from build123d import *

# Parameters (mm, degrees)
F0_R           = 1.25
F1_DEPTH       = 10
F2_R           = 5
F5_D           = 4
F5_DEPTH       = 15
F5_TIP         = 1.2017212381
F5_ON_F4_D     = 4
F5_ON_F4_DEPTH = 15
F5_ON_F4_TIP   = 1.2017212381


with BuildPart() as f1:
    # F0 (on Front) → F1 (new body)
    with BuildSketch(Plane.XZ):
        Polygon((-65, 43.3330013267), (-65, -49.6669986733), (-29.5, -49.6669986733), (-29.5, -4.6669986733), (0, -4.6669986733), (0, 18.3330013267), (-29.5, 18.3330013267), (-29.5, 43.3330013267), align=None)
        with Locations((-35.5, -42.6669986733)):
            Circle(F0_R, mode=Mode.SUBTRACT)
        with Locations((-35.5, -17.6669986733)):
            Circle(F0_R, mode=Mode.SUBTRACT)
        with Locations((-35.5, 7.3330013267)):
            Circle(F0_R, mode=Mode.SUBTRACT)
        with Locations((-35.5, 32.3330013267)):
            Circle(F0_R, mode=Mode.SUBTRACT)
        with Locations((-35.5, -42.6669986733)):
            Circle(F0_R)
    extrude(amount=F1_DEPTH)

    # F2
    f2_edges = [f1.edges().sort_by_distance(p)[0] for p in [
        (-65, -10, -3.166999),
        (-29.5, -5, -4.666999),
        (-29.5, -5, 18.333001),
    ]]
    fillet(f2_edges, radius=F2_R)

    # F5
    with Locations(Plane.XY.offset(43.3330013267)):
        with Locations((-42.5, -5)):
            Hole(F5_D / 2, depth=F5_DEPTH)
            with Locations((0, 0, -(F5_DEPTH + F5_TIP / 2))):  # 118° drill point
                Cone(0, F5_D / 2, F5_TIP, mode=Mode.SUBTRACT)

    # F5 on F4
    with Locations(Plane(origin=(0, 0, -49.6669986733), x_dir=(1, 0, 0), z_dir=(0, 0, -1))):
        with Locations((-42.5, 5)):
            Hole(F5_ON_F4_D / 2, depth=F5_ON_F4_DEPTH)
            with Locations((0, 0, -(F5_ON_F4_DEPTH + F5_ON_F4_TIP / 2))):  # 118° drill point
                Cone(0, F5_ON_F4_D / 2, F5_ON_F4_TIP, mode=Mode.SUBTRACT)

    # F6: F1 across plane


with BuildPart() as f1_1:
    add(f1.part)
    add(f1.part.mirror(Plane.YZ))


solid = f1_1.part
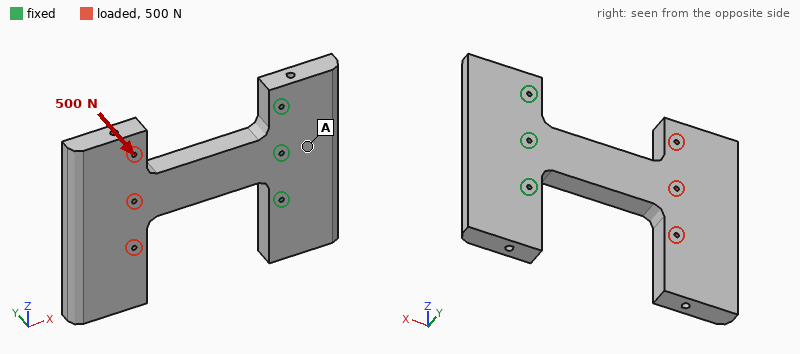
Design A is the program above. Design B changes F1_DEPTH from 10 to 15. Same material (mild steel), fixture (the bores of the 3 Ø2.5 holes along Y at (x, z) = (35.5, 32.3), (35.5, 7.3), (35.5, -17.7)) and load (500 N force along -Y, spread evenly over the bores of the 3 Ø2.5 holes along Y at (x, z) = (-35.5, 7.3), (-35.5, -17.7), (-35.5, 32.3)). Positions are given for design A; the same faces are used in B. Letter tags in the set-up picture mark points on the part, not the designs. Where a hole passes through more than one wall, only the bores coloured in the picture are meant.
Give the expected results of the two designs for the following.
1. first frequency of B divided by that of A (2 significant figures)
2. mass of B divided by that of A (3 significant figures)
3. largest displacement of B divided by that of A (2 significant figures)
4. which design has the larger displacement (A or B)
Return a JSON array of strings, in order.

["1.5", "1.51", "0.31", "A"]
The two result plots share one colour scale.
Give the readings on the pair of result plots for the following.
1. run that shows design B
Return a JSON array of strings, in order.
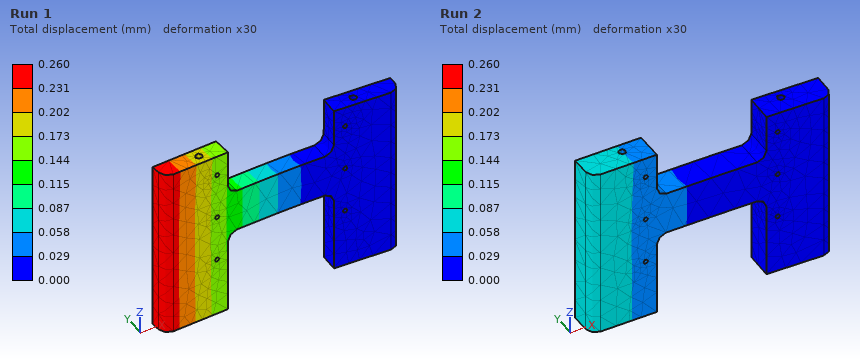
["Run 2"]
